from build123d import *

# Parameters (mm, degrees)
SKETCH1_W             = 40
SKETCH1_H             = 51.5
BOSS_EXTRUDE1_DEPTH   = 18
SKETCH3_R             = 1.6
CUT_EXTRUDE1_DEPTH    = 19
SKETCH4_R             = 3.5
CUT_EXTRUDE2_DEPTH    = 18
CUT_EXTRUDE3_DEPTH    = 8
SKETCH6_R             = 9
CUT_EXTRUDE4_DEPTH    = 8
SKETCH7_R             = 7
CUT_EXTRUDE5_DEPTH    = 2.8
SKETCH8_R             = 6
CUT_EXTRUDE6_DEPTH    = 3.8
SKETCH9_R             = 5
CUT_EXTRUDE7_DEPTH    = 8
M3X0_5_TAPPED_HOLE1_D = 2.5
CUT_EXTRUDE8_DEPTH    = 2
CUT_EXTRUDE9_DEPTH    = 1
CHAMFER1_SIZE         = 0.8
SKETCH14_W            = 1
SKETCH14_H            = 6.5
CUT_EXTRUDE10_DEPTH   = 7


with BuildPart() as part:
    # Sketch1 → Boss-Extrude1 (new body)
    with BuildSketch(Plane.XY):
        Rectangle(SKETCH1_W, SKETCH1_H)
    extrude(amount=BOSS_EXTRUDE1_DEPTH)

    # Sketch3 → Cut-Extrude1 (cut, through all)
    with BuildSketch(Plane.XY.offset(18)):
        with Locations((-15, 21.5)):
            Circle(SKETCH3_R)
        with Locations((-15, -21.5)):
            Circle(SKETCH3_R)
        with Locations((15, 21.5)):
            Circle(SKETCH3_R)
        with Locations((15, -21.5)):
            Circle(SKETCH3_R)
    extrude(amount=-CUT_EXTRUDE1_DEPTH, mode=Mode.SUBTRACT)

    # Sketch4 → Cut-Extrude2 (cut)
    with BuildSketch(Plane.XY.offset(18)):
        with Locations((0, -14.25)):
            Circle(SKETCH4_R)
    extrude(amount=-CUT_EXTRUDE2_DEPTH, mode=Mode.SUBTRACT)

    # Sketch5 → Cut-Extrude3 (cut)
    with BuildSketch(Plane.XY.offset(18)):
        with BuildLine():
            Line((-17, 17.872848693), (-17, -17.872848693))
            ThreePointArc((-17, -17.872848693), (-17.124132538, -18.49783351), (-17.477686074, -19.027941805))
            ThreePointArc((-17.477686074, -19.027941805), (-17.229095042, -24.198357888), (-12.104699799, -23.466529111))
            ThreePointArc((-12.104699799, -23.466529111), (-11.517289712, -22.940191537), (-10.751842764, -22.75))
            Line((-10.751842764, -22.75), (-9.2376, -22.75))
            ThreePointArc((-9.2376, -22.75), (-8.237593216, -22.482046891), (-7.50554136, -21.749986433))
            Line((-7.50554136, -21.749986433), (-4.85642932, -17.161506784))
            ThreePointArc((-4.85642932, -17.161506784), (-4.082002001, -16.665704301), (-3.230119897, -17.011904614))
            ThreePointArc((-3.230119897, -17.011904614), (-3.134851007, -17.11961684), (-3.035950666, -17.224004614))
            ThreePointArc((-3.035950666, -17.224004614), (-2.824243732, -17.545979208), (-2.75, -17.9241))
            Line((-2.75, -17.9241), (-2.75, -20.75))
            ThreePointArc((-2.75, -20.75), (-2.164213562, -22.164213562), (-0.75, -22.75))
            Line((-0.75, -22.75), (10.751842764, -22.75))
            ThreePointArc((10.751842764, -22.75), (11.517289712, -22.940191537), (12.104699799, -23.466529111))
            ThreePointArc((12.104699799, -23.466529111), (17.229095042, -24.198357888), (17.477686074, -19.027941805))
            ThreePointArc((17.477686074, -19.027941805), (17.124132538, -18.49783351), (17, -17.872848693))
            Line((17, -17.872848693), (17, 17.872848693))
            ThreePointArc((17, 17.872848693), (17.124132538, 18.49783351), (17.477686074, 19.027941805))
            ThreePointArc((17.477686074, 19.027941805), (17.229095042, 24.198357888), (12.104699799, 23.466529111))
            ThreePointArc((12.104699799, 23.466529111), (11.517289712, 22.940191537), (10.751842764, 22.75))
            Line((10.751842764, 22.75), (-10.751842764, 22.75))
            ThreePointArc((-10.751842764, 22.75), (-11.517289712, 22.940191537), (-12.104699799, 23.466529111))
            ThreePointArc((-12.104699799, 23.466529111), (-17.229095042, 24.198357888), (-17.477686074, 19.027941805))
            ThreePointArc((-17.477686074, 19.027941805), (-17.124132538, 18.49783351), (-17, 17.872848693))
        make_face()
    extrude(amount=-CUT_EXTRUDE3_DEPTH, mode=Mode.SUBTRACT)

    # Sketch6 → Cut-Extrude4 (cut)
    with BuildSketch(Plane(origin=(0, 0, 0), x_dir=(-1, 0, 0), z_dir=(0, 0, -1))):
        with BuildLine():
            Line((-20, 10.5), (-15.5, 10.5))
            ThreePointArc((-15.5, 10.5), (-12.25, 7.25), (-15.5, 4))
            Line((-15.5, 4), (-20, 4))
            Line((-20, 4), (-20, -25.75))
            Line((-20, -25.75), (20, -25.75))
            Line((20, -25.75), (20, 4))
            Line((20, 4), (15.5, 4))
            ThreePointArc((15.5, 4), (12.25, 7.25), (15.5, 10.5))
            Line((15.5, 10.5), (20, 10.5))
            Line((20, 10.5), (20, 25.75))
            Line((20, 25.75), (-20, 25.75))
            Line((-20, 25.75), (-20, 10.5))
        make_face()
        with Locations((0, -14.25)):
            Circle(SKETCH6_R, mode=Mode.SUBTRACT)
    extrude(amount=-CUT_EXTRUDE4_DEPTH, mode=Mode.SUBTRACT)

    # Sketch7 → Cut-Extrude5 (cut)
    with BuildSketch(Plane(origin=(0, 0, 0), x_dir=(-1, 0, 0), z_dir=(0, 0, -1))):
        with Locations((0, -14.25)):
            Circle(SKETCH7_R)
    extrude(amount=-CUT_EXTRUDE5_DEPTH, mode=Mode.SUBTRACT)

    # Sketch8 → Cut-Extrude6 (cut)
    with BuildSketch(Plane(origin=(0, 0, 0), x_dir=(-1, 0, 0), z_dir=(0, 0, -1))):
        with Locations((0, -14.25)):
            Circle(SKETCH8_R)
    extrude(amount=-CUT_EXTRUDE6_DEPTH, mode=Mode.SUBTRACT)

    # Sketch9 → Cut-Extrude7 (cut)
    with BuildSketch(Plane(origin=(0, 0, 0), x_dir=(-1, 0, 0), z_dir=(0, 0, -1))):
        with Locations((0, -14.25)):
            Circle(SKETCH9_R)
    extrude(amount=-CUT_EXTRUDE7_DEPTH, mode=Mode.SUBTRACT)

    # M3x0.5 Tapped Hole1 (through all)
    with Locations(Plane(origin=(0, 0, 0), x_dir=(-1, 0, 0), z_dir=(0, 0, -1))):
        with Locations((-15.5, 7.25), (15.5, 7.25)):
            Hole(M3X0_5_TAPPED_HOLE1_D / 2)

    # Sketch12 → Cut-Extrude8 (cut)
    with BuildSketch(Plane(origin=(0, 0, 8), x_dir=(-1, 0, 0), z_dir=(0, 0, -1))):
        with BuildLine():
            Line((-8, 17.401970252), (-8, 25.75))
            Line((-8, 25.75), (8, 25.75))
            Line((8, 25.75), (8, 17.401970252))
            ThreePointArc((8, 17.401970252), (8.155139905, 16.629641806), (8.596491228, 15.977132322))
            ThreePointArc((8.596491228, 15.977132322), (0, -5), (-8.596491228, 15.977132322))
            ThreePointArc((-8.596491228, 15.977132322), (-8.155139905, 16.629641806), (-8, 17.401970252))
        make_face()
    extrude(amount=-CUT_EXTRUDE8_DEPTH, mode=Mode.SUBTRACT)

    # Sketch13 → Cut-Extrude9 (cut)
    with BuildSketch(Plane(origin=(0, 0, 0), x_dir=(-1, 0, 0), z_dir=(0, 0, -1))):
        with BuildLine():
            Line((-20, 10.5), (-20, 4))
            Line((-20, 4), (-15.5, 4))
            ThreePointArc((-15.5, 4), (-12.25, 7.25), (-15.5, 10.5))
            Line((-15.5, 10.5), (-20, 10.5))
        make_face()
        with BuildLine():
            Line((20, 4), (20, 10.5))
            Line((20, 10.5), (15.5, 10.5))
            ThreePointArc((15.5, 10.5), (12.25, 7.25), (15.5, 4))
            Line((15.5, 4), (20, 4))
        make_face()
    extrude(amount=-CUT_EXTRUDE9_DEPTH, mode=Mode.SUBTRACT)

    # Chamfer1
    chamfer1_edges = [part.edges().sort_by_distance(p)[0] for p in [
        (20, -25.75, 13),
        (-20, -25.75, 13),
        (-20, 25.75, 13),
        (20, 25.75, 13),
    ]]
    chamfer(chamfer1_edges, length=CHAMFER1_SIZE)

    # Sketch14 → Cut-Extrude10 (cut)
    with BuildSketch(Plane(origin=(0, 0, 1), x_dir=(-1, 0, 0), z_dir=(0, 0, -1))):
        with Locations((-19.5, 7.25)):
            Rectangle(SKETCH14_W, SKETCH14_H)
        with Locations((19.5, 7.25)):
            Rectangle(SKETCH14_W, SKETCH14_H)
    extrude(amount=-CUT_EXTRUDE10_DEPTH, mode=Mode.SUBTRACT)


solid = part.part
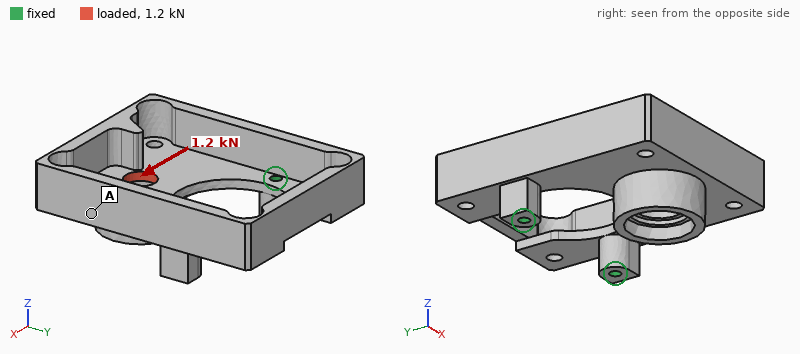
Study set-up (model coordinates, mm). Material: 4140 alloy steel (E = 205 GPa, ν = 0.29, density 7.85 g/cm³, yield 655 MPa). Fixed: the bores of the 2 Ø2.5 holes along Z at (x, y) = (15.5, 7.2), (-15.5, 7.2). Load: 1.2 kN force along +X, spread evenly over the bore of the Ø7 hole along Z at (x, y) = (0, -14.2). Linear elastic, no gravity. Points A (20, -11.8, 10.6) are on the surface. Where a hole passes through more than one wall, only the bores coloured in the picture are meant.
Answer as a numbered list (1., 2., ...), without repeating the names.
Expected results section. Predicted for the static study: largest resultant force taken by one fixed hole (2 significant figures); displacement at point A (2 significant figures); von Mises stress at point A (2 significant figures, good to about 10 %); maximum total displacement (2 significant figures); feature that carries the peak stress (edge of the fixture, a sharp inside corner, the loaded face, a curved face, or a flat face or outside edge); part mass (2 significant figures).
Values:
1. 880 N
2. 12 µm
3. 12 MPa
4. 17 µm
5. edge of the fixture
6. 64 g
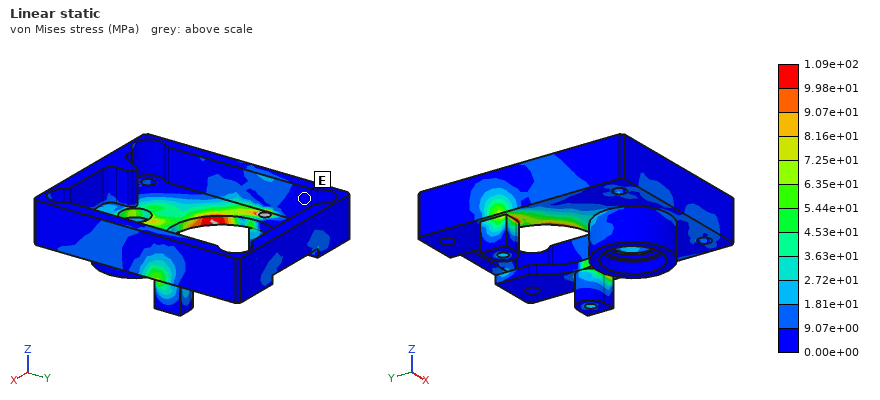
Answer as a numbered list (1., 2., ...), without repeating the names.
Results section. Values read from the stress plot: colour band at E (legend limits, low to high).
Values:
1. 0.00e+00 to 9.07e+00 MPa
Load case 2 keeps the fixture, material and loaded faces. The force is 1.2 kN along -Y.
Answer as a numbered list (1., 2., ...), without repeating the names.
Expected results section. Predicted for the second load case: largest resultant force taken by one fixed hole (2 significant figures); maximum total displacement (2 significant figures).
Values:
1. 630 N
2. 5.3 µm
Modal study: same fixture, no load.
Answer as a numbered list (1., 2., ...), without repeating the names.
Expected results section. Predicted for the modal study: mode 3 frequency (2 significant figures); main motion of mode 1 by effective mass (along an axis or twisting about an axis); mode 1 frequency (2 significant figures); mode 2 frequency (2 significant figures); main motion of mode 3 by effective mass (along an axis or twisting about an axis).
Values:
1. 7300 Hz
2. along Z
3. 2500 Hz
4. 4600 Hz
5. along X
